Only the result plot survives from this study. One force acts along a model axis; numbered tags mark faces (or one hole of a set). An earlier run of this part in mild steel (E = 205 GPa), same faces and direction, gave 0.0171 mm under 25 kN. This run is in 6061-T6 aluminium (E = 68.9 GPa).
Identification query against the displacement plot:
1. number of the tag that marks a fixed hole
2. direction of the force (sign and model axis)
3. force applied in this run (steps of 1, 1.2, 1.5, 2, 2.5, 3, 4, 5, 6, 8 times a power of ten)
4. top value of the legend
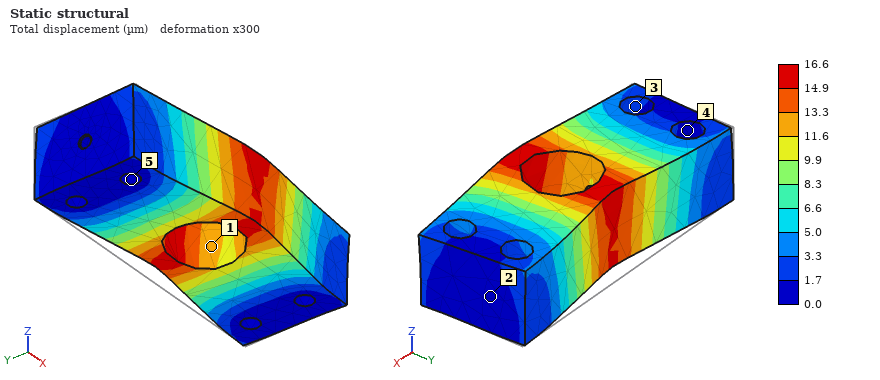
5
-Y
8 kN
16.6 µm
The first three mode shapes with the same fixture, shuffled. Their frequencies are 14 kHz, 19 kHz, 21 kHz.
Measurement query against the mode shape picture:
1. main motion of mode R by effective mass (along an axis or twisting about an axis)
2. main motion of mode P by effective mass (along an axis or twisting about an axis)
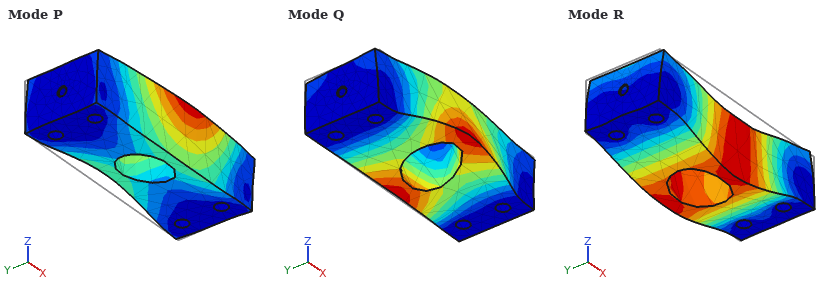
along Z
along Y
